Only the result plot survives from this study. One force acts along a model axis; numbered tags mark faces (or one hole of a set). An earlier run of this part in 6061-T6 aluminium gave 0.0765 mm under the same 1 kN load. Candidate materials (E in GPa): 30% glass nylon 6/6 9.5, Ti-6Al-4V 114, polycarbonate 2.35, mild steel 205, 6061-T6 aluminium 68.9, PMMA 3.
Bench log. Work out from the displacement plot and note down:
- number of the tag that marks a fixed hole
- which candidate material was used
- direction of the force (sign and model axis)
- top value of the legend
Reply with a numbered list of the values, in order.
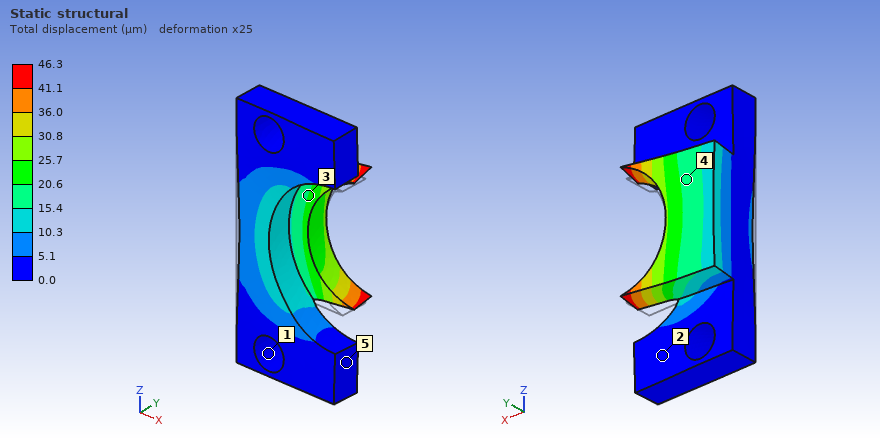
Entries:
1. 1
2. Ti-6Al-4V
3. +Y
4. 46.3 µm
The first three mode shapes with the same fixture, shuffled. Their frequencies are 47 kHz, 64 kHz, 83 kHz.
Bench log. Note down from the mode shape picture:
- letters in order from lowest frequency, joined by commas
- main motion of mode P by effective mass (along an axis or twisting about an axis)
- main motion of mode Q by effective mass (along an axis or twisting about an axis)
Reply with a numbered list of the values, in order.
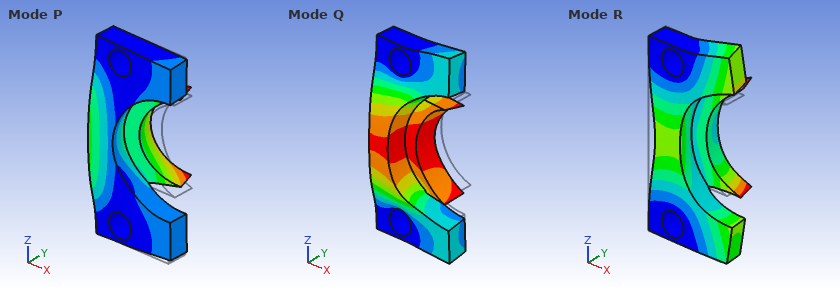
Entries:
1. P, Q, R
2. along X
3. along Y
